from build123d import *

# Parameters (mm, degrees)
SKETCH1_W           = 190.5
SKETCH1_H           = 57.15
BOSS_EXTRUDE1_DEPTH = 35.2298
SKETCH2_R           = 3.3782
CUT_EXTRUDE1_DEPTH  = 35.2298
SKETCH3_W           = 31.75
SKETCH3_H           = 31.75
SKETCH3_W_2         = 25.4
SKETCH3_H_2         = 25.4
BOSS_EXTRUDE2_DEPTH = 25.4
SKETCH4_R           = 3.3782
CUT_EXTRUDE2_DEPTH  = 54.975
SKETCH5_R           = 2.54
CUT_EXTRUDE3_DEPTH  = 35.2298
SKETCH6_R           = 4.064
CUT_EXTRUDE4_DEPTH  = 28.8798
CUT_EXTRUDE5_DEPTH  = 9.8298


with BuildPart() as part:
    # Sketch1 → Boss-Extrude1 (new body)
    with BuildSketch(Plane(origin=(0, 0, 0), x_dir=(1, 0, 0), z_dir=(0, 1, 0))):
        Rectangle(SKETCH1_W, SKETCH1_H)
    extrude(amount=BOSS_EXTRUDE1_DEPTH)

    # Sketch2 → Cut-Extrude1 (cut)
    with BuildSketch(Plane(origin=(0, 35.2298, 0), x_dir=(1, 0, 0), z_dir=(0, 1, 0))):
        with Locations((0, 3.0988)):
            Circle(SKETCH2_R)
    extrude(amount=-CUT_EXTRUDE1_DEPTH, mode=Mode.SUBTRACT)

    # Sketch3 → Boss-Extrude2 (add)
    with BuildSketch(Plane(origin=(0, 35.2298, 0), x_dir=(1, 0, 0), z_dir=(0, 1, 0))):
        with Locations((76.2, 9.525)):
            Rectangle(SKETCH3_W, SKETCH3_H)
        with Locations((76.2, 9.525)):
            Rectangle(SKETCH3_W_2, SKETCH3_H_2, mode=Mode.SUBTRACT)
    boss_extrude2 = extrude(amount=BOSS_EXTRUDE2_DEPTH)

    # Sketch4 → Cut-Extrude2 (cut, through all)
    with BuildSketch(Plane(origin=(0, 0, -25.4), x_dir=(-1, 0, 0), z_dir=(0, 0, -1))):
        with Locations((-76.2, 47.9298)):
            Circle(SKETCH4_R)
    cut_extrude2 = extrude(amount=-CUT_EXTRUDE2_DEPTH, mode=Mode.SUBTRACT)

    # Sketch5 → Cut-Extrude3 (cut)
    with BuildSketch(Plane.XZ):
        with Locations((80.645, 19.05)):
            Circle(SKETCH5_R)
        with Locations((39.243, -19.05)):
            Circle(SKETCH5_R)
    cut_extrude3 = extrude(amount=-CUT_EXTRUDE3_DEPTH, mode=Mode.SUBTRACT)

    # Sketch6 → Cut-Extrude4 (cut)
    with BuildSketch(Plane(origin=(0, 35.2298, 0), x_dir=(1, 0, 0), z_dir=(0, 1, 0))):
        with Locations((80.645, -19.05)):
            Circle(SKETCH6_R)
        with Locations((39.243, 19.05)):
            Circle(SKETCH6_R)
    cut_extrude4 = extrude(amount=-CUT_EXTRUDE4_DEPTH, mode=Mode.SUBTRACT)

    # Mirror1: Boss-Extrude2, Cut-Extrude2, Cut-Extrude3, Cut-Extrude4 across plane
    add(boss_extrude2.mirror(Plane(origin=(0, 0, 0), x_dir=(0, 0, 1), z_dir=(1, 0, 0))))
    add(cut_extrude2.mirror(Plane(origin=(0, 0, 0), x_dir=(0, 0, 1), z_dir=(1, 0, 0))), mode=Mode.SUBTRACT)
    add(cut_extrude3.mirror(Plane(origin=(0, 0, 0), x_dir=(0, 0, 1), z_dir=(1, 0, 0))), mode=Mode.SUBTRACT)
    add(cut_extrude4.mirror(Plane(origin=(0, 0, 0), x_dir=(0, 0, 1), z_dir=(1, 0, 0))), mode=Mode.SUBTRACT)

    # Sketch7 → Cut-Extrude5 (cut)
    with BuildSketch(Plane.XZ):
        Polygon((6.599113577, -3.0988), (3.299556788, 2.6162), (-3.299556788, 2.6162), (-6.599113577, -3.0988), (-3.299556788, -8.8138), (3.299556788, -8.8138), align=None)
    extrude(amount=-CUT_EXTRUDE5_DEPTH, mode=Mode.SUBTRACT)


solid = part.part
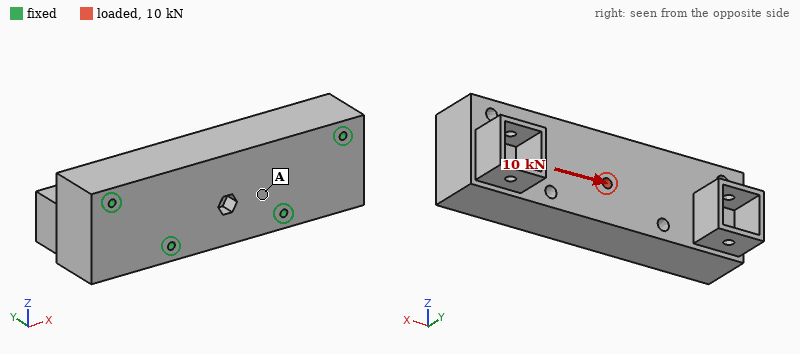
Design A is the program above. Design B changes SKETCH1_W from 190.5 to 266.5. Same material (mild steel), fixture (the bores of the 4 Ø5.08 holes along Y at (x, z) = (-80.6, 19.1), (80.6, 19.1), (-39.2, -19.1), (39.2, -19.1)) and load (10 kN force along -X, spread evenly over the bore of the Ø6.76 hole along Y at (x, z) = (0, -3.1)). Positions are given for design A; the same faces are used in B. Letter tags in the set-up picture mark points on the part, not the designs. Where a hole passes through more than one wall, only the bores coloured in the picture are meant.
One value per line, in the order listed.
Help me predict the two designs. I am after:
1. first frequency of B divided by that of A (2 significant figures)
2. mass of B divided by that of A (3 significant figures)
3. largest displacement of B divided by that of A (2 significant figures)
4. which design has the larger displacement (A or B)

0.73
1.39
1.2
B
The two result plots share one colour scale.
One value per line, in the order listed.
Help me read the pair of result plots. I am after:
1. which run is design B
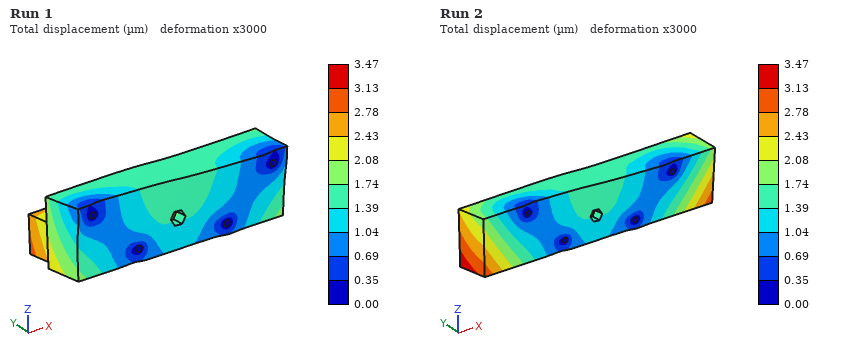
Run 2
